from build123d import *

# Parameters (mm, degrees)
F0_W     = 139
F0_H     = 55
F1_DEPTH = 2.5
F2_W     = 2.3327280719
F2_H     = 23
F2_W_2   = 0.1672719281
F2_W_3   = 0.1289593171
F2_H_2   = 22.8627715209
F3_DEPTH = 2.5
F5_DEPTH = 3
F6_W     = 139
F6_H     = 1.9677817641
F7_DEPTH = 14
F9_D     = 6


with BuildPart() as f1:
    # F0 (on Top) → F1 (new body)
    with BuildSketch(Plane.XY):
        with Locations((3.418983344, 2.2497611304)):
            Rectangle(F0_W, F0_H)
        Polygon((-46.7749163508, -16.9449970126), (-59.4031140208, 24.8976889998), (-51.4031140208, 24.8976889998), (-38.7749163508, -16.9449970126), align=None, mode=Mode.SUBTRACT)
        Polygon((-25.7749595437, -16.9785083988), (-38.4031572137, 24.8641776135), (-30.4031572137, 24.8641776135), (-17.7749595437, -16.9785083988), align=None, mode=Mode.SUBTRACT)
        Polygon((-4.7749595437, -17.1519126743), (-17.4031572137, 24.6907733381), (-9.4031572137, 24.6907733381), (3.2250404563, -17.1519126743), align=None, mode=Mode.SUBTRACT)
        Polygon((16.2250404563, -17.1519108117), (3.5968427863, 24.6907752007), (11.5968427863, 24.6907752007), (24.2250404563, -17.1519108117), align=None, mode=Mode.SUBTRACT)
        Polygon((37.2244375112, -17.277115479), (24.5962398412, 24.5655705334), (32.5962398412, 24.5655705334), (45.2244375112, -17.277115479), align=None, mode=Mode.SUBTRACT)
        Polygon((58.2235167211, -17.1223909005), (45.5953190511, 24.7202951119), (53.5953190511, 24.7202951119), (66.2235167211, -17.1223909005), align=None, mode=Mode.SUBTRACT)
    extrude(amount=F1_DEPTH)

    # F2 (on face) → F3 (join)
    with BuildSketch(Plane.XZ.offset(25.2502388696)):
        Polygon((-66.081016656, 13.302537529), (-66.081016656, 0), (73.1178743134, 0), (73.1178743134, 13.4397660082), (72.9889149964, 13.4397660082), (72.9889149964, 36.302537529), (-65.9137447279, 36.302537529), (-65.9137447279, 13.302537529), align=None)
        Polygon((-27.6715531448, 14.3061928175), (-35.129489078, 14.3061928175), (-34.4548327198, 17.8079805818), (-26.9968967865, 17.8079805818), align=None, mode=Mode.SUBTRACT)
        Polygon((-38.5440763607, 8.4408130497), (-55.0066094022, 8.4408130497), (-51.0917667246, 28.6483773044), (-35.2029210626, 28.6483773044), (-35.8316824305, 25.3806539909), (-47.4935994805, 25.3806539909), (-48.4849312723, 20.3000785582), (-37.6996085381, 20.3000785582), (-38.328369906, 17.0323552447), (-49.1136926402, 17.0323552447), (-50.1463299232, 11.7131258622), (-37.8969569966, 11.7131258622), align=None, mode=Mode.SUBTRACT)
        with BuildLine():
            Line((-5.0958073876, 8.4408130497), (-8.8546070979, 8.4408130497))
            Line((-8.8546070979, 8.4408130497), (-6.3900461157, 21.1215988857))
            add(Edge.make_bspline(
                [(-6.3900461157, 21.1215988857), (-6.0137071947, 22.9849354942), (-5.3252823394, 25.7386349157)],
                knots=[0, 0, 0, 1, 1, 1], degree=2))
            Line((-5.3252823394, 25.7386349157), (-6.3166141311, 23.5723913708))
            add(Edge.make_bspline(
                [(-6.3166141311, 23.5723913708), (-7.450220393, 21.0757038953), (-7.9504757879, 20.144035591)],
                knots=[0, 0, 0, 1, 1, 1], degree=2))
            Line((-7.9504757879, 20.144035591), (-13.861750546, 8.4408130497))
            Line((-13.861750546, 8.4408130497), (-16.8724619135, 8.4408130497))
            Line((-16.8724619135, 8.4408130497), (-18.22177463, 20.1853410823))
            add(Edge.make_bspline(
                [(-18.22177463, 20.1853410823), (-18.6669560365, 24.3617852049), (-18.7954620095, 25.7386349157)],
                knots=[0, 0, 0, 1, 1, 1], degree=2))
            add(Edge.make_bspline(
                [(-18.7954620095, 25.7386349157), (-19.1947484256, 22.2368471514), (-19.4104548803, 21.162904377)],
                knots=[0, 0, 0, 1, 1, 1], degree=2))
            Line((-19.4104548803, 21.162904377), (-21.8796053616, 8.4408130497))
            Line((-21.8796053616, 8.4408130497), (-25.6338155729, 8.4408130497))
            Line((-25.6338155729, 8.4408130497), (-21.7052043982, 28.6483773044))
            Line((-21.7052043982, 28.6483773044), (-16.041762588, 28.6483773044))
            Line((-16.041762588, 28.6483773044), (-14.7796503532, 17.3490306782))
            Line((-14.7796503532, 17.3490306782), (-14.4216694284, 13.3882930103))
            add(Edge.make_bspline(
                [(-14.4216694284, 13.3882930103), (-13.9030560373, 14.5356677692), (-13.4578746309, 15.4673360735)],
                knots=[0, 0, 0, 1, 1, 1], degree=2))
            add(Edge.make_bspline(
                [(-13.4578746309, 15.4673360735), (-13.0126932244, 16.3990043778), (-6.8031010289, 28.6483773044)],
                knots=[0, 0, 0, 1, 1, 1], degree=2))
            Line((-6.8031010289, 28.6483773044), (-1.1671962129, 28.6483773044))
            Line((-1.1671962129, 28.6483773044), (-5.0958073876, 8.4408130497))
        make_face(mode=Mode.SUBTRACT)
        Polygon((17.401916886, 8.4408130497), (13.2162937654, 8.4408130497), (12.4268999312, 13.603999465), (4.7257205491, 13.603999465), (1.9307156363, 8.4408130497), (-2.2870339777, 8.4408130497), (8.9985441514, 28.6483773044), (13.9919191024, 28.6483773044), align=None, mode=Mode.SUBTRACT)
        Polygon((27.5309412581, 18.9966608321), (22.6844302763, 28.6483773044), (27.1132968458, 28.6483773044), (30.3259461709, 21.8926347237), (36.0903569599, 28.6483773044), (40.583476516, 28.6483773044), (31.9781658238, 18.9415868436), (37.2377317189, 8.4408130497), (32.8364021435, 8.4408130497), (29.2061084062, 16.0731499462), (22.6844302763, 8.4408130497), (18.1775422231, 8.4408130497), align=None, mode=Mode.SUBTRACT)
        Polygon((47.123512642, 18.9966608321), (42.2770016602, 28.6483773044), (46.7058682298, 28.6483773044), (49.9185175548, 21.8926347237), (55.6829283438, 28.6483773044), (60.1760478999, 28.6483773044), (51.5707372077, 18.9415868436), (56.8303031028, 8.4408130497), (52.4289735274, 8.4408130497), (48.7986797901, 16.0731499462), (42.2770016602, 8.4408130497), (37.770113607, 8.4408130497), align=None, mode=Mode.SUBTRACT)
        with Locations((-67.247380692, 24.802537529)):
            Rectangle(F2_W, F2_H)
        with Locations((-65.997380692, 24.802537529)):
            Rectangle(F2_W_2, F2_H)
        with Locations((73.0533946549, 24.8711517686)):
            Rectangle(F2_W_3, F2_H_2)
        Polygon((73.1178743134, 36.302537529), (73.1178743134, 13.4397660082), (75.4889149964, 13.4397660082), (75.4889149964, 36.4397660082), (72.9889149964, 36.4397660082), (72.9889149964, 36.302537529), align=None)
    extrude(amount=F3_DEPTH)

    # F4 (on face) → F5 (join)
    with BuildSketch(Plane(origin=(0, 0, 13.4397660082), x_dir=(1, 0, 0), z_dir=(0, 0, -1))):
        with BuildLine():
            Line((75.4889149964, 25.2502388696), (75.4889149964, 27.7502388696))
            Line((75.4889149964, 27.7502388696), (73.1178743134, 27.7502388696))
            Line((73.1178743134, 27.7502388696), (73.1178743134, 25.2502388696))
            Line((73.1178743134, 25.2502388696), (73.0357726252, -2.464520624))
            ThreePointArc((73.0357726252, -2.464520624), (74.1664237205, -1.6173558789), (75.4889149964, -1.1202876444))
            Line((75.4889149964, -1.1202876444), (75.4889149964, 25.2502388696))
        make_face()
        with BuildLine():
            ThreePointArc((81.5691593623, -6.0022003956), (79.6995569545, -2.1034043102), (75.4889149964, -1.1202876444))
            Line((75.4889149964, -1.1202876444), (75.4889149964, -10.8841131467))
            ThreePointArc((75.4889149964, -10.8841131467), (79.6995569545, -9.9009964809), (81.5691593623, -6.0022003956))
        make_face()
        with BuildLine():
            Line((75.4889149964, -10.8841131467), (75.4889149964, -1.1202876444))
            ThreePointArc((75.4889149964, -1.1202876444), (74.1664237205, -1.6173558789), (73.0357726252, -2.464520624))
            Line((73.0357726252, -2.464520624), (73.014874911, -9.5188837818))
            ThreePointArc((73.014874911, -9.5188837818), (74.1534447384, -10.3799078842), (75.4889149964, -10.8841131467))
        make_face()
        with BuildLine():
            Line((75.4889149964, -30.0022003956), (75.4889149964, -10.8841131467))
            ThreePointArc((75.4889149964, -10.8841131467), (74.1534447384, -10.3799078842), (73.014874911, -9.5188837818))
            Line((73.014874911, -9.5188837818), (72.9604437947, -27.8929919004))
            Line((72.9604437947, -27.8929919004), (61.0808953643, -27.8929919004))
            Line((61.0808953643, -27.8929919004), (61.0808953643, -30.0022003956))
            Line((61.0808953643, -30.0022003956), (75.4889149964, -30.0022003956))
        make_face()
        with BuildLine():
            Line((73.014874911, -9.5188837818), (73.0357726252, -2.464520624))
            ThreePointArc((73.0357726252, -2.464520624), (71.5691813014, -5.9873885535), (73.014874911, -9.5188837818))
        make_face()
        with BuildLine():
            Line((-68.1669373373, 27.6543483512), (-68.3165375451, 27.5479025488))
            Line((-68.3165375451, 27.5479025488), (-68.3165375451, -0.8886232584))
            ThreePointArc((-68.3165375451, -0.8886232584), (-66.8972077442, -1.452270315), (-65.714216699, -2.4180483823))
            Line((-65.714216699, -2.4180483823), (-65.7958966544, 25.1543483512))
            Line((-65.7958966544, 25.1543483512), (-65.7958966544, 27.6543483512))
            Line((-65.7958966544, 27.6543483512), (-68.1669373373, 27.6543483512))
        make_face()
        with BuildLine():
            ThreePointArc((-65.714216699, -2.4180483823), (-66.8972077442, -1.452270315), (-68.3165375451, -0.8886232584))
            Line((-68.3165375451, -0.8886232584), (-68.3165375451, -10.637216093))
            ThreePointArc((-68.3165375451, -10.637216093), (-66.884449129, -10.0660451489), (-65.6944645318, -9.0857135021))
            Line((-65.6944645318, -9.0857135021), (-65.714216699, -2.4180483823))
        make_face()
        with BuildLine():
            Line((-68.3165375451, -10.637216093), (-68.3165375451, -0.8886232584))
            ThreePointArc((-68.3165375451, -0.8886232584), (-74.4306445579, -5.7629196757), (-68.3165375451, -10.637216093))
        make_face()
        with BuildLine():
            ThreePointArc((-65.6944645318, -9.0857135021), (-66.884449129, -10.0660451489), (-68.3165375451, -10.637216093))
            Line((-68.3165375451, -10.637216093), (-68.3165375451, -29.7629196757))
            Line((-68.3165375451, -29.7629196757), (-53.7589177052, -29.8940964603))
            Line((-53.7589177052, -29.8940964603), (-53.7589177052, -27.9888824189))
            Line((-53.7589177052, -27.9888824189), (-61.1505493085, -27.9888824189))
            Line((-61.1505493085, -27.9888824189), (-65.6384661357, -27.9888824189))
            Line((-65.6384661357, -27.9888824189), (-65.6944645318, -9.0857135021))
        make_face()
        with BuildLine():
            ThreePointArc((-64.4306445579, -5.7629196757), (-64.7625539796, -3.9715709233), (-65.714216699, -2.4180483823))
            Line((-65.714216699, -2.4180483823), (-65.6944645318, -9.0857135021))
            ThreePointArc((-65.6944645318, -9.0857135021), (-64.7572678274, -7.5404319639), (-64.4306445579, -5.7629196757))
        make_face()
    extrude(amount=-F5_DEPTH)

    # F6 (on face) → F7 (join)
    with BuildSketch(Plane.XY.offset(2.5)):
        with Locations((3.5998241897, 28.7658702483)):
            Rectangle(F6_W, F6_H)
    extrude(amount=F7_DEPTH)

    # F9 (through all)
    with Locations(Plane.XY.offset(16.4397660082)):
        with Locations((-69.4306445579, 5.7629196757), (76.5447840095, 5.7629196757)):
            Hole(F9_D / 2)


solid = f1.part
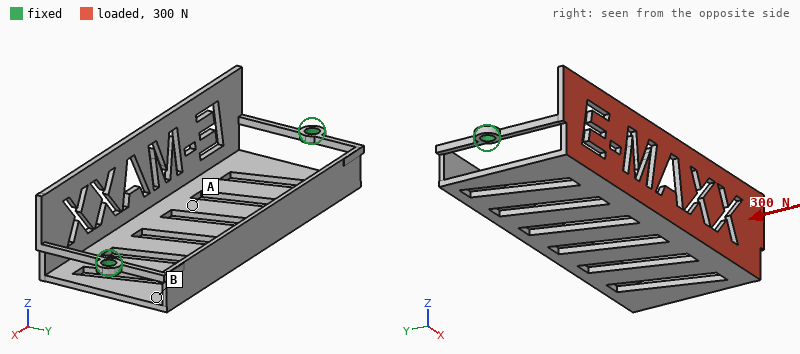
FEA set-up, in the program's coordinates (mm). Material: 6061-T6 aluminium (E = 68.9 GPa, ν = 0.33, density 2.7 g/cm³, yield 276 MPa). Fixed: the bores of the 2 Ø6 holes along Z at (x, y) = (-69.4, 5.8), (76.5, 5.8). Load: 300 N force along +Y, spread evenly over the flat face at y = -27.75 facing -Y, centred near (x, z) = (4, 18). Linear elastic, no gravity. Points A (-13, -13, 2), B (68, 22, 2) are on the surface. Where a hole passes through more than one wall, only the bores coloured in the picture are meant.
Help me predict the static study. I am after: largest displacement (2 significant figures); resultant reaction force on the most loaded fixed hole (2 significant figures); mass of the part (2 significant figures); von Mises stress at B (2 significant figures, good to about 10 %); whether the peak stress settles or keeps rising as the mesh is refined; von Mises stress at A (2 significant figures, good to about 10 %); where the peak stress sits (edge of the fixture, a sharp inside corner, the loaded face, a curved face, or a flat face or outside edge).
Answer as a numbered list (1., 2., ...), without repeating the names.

1. 0.64 mm
2. 150 N
3. 79 g
4. 9.7 MPa
5. keeps rising
6. 23 MPa
7. a sharp inside corner
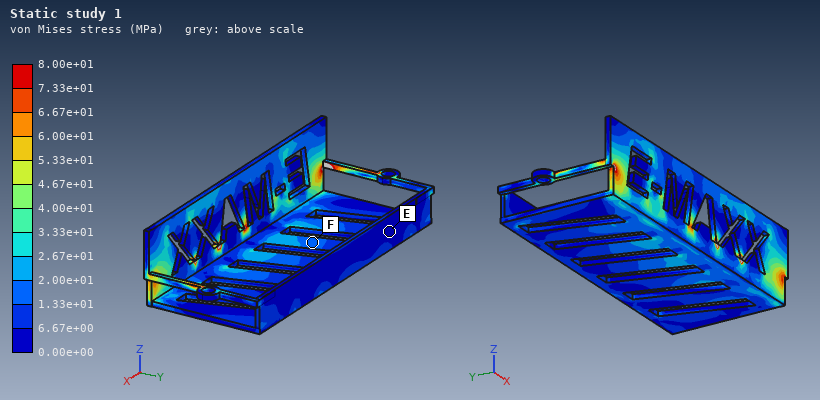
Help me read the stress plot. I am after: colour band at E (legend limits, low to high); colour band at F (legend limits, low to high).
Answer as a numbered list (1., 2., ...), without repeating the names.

1. 0.00e+00 to 6.67e+00 MPa
2. 1.33e+01 to 2.00e+01 MPa
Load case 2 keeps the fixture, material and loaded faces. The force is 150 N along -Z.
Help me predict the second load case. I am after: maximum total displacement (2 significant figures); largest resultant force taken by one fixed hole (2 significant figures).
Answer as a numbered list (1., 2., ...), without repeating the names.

1. 1.1 mm
2. 76 N
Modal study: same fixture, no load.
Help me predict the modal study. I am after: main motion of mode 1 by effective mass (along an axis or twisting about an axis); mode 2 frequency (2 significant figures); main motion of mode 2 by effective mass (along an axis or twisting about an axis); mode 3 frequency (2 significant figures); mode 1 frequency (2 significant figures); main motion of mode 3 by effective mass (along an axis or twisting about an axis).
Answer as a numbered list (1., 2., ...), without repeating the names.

1. along Z
2. 470 Hz
3. along X
4. 600 Hz
5. 300 Hz
6. along Z
